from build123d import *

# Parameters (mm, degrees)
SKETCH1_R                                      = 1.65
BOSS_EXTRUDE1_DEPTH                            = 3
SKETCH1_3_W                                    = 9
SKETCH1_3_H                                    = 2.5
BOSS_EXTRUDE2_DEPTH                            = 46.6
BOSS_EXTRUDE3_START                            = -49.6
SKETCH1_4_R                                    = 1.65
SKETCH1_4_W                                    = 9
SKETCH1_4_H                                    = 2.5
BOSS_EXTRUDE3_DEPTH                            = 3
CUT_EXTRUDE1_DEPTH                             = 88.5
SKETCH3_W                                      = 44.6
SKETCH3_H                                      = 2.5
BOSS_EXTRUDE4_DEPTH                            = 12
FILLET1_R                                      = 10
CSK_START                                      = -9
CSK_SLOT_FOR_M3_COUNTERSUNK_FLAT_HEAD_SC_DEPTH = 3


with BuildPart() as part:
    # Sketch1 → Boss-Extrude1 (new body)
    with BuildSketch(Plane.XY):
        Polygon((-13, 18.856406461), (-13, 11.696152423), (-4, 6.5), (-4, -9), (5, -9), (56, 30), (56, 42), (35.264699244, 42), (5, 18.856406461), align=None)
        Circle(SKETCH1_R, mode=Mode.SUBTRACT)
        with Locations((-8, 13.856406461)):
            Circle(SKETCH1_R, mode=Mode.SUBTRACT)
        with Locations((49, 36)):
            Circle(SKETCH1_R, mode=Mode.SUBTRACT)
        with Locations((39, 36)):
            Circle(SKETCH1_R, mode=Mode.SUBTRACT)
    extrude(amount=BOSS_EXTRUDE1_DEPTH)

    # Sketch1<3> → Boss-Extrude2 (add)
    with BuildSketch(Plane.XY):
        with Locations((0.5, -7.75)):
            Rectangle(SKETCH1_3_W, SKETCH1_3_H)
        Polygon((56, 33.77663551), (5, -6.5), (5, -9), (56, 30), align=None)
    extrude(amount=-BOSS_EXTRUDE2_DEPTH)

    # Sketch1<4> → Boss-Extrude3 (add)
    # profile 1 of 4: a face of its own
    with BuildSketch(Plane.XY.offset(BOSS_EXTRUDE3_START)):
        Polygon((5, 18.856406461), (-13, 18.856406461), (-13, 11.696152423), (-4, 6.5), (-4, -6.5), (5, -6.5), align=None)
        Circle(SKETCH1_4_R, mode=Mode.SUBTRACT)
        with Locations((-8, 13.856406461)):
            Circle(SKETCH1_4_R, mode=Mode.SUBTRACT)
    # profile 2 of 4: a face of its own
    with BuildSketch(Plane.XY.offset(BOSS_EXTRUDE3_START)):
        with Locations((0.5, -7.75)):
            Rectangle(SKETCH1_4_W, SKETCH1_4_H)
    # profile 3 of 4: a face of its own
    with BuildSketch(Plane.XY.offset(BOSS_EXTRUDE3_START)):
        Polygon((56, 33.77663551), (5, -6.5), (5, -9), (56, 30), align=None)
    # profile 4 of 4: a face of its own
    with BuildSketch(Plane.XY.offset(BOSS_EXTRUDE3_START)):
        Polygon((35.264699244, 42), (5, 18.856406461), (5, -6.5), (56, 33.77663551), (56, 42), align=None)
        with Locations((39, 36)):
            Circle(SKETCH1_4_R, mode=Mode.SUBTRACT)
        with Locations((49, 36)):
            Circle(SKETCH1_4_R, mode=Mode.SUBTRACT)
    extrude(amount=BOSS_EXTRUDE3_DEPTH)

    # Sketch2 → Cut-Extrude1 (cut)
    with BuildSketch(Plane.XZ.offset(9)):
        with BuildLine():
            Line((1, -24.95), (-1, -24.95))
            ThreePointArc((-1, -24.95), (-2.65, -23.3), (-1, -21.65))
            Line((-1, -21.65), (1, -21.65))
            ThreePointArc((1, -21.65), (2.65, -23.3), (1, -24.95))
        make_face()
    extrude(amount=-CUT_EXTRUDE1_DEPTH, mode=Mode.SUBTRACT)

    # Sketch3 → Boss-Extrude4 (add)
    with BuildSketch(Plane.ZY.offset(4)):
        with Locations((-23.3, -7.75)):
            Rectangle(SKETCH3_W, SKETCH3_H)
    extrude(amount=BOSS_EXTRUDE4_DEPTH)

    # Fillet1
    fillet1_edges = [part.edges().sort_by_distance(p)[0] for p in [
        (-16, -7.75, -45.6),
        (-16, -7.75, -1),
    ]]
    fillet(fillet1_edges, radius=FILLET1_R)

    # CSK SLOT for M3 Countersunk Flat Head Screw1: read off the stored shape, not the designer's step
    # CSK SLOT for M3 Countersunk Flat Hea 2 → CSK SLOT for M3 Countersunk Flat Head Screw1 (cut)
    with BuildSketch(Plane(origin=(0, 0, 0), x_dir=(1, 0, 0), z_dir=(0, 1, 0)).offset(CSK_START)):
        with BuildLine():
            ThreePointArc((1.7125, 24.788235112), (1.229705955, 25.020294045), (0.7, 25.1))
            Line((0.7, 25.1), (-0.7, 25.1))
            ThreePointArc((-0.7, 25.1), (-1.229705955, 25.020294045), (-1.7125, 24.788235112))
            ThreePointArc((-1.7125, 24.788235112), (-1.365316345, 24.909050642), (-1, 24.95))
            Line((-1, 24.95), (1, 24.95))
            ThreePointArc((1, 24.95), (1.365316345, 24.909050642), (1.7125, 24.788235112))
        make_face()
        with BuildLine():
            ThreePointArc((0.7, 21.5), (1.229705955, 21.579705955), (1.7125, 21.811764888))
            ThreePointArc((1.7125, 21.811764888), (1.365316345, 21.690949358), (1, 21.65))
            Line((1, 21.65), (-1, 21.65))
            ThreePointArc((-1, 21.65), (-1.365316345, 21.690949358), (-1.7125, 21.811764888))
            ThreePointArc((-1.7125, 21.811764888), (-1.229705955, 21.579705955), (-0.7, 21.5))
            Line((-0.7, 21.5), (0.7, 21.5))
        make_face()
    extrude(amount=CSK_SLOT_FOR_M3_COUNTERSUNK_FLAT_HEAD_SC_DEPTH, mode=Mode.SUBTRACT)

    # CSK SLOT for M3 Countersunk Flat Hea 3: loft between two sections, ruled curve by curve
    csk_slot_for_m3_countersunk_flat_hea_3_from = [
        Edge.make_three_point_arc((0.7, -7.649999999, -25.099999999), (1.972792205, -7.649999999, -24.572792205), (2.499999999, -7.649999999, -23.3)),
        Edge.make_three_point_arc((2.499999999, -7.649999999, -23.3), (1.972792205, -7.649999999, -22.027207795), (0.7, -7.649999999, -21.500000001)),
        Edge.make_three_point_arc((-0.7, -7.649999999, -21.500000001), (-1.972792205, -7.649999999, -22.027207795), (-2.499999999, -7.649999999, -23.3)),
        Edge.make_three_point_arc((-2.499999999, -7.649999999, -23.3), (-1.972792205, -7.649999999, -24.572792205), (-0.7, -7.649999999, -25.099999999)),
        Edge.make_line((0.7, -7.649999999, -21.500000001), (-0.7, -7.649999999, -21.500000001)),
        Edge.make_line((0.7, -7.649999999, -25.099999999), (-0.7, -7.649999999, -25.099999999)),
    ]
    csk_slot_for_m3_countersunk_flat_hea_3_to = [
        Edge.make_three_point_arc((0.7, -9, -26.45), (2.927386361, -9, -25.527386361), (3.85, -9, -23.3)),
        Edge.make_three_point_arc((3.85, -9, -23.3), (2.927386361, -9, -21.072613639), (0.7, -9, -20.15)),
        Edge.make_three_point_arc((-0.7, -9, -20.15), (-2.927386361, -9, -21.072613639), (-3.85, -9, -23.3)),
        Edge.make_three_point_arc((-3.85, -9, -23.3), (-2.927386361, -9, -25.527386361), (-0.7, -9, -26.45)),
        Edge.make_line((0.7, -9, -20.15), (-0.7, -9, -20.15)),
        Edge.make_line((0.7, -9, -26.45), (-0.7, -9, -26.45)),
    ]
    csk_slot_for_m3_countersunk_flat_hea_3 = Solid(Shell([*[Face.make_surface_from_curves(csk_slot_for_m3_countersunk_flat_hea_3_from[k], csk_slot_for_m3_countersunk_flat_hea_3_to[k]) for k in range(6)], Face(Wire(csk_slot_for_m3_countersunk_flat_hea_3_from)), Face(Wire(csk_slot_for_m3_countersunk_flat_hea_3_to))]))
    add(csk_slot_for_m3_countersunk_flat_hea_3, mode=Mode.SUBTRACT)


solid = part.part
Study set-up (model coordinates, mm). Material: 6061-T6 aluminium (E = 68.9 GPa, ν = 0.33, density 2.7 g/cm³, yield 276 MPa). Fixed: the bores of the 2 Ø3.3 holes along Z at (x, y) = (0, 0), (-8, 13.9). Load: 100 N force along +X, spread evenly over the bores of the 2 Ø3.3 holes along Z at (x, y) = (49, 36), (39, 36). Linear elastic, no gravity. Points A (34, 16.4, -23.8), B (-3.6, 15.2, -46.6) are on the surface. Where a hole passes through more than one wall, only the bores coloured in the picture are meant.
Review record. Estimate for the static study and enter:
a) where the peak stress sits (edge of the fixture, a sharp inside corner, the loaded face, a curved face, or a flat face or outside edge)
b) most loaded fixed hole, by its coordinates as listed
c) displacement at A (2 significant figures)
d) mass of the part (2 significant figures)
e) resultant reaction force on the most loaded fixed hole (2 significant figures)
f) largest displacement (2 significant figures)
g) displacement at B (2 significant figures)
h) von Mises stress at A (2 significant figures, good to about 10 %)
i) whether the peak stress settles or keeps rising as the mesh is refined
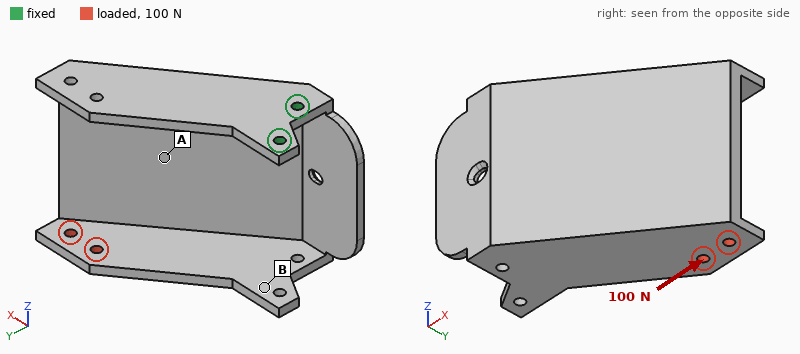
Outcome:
edge of the fixture
(-8, 13.9)
0.44 mm
51 g
250 N
1.2 mm
0.66 mm
28 MPa
keeps rising
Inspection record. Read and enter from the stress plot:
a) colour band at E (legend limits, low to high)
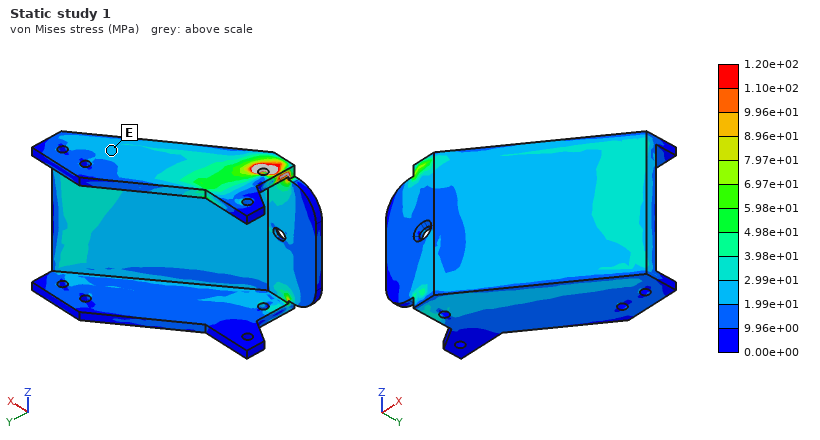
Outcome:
1.99e+01 to 2.99e+01 MPa
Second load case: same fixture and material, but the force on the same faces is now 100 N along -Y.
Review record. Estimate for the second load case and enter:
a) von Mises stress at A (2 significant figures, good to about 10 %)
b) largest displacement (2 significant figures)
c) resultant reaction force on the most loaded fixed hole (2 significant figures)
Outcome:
18 MPa
1.1 mm
300 N
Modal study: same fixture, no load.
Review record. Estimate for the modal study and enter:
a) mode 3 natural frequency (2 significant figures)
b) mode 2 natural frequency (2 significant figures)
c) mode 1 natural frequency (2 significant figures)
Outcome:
930 Hz
410 Hz
390 Hz
